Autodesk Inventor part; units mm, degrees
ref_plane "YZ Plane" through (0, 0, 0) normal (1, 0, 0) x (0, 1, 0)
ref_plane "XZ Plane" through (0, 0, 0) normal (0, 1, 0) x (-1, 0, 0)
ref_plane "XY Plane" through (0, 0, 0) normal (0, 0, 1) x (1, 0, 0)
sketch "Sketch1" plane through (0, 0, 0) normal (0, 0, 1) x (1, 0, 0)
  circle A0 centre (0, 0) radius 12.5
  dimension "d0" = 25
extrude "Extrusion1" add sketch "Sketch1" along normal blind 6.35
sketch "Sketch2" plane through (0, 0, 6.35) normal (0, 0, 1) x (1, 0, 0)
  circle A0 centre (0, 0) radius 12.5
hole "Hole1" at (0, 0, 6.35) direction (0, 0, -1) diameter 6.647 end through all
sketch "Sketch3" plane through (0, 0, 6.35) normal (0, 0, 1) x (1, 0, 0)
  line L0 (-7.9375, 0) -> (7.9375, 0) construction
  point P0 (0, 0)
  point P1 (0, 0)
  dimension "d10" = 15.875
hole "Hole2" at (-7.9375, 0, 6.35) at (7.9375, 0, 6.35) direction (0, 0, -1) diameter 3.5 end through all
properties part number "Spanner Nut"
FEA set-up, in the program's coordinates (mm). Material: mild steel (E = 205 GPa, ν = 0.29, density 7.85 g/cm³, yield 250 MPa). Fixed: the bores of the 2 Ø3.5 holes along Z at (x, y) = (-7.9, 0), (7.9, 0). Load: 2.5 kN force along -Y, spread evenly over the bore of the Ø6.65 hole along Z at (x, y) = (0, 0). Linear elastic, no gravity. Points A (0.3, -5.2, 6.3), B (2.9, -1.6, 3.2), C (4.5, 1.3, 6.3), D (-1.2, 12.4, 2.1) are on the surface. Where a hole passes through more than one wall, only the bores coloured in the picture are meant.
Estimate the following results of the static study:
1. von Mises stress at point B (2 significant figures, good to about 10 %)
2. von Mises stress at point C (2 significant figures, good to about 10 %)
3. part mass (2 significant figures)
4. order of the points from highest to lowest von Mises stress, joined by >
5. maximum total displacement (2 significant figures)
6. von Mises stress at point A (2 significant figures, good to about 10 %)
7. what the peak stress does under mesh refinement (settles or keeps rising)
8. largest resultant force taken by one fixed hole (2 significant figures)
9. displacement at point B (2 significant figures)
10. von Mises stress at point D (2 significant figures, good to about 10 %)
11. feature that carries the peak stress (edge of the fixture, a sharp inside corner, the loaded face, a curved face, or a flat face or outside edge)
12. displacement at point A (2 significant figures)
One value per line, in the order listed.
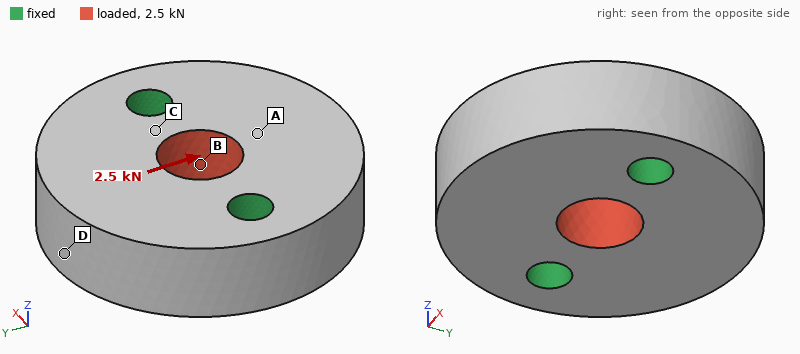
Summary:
33 MPa
25 MPa
22 g
B > C > A > D
1.1 µm
17 MPa
keeps rising
1.3 kN
0.86 µm
9.2 MPa
edge of the fixture
0.89 µm
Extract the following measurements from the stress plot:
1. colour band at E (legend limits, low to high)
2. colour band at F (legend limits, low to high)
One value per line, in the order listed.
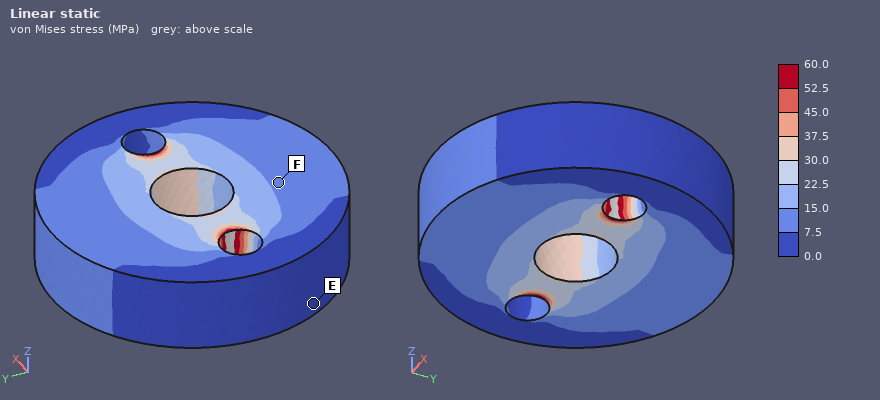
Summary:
0.0 to 7.5 MPa
7.5 to 15.0 MPa
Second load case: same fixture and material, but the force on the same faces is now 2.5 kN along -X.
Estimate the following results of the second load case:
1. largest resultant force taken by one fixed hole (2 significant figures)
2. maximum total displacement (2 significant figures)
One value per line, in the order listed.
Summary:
1.3 kN
0.82 µm
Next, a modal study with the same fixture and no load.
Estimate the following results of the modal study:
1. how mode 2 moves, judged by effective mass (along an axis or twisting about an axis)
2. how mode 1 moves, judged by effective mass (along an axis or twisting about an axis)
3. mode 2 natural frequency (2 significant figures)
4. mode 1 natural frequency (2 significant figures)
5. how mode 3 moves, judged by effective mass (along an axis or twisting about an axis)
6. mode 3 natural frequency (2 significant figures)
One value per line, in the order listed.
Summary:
along Z
twisting about X
35 kHz
31 kHz
twisting about Z
61 kHz
